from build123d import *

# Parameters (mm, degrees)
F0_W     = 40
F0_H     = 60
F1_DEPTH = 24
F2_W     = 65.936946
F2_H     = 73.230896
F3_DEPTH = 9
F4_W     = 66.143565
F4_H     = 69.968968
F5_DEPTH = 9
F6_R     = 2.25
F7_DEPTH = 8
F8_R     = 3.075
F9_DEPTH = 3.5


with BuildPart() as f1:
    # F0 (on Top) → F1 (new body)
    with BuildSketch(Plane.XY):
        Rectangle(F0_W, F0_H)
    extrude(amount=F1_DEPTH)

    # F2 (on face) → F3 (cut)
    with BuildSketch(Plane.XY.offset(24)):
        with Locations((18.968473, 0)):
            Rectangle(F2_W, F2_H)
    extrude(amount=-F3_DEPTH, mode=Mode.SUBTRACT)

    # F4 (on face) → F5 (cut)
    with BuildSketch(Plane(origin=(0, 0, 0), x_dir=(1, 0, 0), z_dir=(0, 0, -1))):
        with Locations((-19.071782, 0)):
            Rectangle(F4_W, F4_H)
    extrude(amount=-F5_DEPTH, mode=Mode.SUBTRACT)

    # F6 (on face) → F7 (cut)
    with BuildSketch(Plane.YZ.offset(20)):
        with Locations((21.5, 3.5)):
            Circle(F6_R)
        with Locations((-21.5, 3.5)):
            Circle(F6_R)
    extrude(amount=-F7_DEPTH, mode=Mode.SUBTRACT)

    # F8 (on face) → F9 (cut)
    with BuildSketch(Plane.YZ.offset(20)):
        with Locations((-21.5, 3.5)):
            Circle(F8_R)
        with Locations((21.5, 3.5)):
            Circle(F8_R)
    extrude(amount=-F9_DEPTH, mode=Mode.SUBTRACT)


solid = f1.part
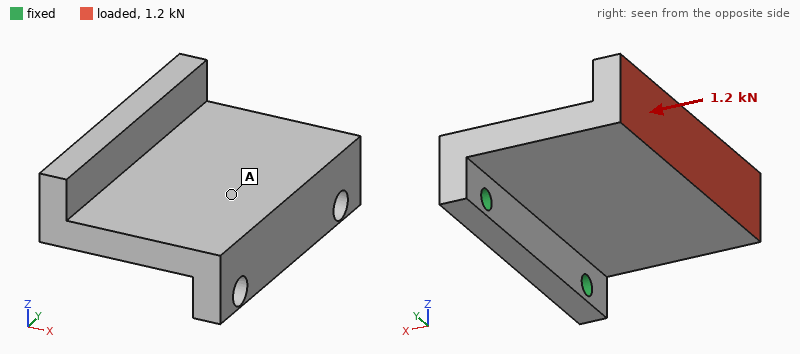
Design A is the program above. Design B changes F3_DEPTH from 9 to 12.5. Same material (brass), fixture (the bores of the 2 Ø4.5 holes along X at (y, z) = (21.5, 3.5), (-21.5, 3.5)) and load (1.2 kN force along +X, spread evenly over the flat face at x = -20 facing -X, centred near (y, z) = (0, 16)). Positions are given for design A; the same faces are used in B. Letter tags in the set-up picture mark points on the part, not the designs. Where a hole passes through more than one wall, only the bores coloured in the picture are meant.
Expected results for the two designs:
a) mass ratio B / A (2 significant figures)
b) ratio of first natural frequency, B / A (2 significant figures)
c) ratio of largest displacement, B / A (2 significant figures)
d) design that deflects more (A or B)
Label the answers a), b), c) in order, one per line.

a) 0.65
b) 0.57
c) 4.3
d) B
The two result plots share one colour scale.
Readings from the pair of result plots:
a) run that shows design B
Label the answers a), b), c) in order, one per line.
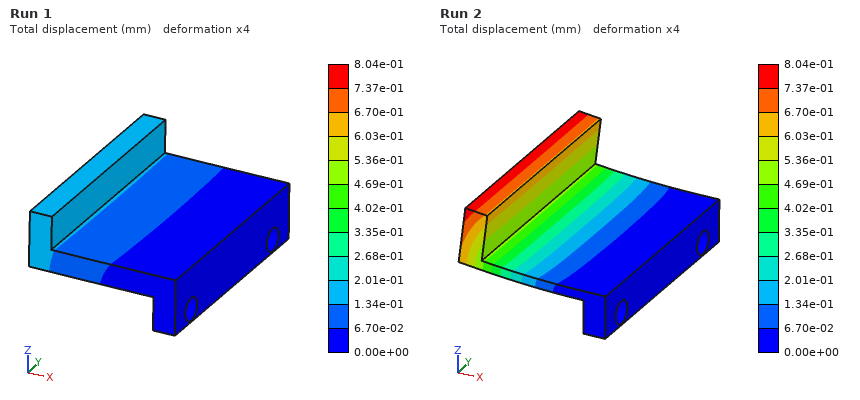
a) Run 2
